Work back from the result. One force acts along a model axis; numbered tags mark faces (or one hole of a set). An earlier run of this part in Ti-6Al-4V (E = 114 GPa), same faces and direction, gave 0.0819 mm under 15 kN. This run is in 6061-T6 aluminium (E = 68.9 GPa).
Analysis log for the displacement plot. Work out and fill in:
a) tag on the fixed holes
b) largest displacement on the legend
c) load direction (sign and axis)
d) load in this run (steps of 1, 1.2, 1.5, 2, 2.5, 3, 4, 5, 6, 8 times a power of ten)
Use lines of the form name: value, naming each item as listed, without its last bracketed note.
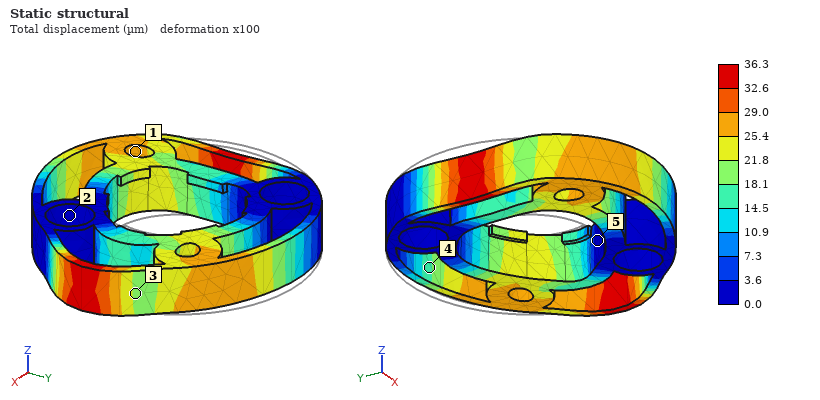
tag on the fixed holes: 2
largest displacement on the legend: 36.3 µm
load direction: -Y
load in this run: 4 kN
